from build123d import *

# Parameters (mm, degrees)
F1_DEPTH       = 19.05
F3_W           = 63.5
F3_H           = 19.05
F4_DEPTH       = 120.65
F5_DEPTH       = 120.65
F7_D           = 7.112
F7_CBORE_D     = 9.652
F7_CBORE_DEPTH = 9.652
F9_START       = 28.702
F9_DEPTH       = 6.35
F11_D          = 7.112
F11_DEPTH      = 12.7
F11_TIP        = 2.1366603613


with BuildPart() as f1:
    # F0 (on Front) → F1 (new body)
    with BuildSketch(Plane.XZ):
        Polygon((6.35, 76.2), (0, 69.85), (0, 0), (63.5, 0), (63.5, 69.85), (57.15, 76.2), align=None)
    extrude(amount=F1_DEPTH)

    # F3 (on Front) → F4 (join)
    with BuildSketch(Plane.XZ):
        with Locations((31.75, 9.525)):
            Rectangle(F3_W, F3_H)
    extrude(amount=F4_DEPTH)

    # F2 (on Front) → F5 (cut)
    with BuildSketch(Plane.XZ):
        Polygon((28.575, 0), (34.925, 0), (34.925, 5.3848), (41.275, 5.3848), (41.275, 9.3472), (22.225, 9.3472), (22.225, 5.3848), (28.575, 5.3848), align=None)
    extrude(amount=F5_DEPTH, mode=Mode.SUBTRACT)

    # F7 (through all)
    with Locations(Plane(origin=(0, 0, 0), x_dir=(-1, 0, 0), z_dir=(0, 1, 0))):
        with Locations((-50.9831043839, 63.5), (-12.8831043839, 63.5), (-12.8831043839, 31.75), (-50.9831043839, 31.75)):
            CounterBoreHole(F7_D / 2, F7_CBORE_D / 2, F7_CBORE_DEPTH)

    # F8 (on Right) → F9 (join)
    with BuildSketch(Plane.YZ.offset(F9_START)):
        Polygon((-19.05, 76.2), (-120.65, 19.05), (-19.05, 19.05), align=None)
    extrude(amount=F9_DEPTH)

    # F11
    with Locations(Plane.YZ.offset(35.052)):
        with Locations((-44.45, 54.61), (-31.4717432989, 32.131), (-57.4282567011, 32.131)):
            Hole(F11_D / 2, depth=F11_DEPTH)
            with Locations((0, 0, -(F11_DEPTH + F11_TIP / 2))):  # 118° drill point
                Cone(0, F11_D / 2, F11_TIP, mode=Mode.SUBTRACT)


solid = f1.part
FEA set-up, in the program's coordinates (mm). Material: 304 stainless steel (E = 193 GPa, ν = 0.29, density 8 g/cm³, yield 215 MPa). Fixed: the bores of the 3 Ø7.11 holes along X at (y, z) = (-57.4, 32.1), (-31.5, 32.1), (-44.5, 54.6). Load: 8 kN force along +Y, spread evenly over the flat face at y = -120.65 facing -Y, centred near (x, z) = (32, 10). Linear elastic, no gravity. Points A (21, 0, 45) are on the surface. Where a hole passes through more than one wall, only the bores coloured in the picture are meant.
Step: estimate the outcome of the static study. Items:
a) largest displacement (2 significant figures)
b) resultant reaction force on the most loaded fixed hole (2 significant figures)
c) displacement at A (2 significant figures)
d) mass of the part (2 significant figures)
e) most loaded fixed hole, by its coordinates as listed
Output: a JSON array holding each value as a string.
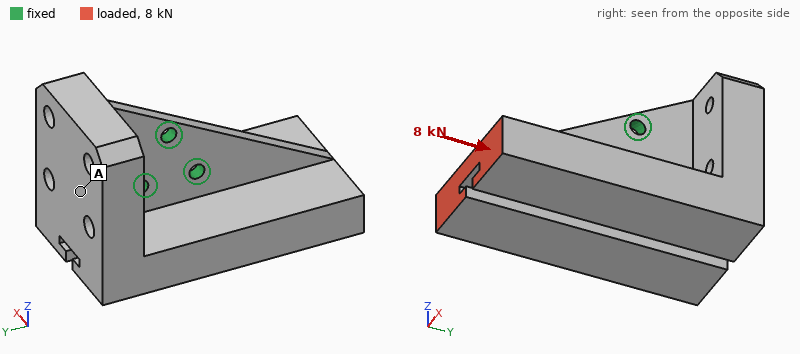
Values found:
["22 µm", "6.8 kN", "6.4 µm", "1.7 kg", "(-31.5, 32.1)"]
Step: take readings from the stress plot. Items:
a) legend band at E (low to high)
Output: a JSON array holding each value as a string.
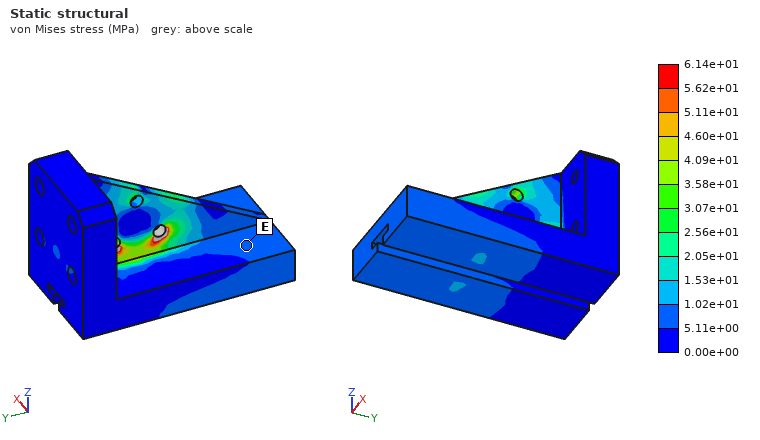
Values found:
["5.11e+00 to 1.02e+01 MPa"]
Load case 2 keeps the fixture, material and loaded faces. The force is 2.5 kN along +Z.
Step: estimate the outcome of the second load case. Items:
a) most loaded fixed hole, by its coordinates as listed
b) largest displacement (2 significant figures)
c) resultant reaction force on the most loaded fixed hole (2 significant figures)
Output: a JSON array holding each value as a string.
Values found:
["(-57.4, 32.1)", "36 µm", "4.8 kN"]
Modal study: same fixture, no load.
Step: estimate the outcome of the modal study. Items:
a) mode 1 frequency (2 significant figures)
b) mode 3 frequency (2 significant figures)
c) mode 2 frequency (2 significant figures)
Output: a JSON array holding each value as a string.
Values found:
["1200 Hz", "2800 Hz", "1500 Hz"]
